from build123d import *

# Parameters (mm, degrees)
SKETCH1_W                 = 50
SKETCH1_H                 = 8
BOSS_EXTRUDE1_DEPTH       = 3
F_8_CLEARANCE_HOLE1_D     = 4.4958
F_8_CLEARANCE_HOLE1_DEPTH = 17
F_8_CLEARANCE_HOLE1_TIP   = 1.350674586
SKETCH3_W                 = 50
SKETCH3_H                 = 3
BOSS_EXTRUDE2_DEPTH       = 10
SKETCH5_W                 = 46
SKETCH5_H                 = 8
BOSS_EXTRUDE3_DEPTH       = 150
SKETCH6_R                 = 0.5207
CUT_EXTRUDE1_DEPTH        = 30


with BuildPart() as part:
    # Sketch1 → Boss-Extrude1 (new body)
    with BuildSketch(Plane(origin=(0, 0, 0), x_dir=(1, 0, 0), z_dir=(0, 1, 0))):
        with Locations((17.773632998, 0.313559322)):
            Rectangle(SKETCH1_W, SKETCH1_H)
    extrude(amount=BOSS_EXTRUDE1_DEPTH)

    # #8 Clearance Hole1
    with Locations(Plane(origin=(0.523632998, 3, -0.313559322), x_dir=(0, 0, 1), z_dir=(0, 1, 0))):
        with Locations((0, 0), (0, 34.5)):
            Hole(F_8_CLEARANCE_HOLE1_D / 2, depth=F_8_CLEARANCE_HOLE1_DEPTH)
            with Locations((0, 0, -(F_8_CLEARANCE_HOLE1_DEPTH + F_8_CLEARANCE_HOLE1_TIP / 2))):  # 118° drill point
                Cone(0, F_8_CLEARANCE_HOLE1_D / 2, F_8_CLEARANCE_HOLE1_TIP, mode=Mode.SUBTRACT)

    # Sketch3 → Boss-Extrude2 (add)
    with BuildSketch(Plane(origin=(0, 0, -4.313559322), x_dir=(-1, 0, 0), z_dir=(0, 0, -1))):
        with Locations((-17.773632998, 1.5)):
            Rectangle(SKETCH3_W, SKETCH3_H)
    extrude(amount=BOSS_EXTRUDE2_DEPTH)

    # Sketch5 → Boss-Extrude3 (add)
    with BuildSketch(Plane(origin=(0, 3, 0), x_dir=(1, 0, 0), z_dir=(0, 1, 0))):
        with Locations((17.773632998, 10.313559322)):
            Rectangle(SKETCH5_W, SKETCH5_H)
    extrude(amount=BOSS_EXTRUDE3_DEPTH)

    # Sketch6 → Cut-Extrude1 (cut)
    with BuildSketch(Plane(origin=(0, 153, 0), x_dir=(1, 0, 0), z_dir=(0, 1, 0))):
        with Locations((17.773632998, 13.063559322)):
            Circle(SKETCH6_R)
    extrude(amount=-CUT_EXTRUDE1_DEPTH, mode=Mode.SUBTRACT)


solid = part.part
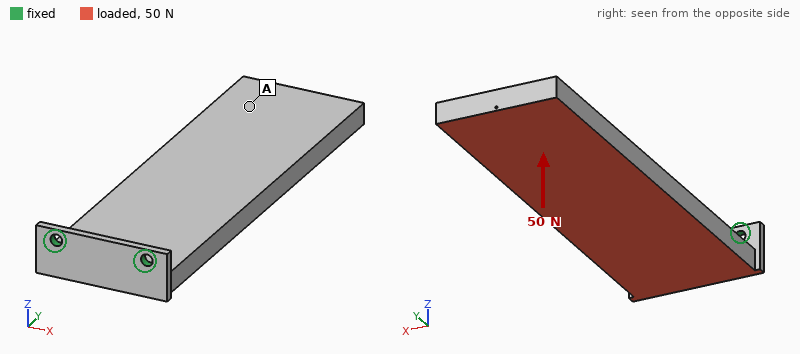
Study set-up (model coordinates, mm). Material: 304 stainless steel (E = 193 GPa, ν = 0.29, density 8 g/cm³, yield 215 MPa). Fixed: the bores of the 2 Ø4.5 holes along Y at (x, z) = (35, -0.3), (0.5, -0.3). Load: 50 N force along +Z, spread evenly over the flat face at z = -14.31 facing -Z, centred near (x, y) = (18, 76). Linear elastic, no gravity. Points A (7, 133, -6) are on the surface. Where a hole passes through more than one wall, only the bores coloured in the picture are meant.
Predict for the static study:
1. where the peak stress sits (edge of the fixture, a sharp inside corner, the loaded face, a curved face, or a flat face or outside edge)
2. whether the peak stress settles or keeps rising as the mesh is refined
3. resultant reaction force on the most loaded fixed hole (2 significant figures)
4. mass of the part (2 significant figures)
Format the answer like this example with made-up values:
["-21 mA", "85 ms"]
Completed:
["edge of the fixture", "keeps rising", "33 N", "460 g"]
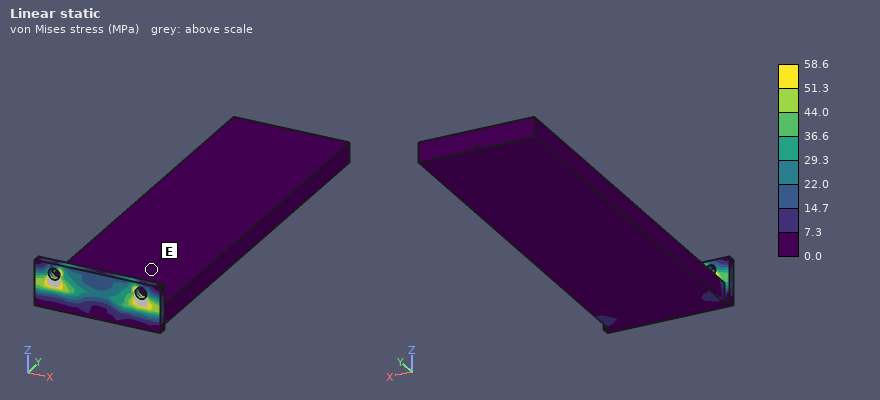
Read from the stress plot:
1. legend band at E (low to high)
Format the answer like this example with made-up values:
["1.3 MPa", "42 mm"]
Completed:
["0.0 to 7.3 MPa"]
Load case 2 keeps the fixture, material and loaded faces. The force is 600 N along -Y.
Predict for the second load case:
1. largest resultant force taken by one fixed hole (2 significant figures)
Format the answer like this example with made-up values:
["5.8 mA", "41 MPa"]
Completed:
["300 N"]
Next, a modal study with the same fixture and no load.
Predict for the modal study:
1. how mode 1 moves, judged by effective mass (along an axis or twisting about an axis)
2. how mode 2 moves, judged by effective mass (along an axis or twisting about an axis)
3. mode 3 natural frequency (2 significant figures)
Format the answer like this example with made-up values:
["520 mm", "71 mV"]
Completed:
["along Z", "along X", "1200 Hz"]
